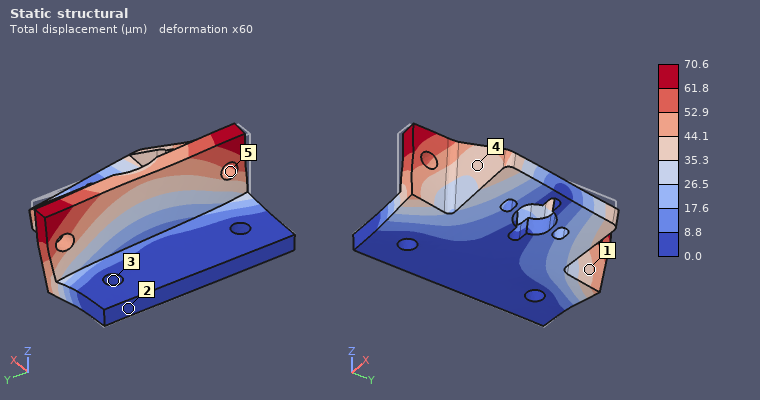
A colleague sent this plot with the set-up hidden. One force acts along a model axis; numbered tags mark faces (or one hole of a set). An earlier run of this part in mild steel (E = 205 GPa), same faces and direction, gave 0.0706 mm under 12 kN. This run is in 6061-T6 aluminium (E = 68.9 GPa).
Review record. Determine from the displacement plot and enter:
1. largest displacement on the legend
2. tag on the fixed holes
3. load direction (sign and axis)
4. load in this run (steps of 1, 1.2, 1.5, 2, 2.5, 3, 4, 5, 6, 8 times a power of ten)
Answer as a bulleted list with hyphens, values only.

- 70.6 µm
- 3
- +Y
- 4 kN
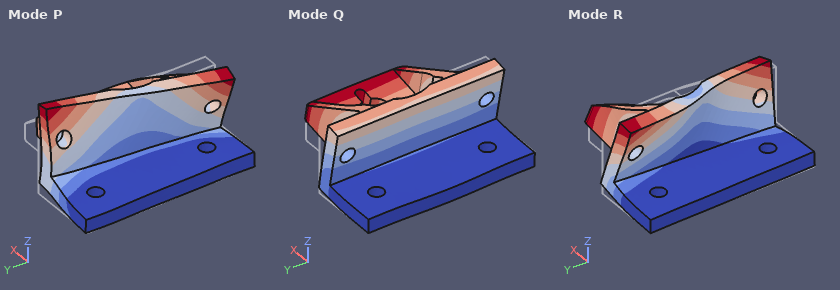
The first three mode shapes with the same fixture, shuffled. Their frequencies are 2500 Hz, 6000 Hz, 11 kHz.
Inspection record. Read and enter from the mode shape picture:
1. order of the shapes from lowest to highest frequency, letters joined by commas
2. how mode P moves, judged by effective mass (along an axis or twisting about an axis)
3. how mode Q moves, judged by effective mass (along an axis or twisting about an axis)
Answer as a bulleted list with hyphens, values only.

- Q, R, P
- along Y
- along Z
